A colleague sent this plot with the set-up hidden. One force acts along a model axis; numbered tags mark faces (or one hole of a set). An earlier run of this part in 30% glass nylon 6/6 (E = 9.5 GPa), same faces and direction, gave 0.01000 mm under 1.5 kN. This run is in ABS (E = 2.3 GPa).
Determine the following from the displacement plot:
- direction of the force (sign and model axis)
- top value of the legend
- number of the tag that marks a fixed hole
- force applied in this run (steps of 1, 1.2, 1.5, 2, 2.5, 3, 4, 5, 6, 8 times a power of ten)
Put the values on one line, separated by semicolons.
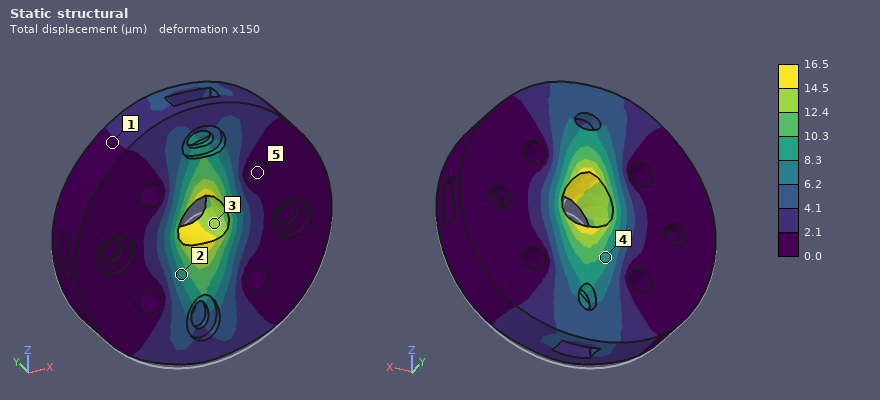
+Z; 16.5 µm; 5; 600 N
